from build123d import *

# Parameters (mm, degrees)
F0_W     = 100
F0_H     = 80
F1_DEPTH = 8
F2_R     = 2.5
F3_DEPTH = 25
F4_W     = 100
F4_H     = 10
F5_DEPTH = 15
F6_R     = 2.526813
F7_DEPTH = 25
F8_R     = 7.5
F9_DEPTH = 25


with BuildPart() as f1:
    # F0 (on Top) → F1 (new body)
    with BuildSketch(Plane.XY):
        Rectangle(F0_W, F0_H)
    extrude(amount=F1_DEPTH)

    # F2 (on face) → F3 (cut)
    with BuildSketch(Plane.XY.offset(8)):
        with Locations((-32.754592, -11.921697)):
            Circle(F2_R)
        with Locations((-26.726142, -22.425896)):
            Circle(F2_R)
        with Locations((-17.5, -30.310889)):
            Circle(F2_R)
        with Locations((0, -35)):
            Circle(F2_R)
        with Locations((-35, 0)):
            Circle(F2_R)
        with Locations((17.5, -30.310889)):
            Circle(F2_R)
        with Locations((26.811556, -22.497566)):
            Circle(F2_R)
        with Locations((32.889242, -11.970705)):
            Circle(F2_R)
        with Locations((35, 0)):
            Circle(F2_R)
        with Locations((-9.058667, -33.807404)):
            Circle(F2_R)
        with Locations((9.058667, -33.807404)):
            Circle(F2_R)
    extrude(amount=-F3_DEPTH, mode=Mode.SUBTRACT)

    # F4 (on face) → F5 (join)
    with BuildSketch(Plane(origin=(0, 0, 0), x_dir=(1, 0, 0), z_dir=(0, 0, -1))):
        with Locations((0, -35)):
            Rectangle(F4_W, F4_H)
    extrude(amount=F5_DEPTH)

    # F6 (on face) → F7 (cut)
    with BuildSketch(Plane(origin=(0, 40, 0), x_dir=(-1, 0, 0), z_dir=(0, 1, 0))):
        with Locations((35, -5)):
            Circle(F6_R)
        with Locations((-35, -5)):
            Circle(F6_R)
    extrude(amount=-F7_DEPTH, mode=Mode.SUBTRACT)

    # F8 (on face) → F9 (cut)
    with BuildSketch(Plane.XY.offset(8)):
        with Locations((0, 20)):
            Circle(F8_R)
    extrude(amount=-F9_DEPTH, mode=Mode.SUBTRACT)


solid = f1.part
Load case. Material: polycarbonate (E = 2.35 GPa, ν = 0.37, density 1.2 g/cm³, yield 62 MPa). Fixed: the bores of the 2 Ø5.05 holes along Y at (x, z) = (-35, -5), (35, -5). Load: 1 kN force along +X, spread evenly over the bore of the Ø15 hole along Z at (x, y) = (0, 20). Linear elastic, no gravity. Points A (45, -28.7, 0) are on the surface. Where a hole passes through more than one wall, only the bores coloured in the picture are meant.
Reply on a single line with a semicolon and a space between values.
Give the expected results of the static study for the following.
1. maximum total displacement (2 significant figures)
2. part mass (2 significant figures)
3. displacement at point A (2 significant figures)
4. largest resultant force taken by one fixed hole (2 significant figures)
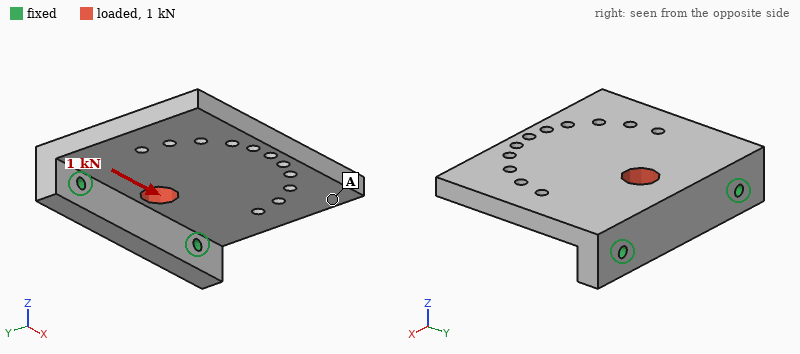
0.11 mm; 91 g; 0.099 mm; 550 N
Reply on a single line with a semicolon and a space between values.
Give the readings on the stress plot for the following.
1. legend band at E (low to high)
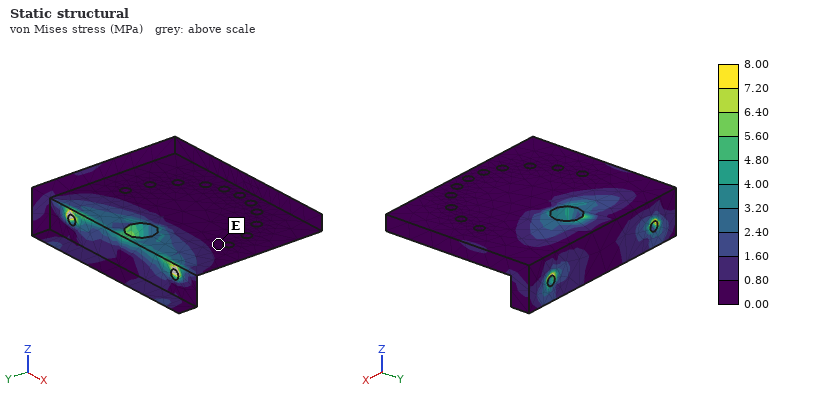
0.00 to 0.80 MPa
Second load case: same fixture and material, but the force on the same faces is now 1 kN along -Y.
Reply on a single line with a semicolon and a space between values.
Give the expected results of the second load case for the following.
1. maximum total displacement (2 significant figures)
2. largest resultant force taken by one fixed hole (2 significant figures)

0.49 mm; 510 N
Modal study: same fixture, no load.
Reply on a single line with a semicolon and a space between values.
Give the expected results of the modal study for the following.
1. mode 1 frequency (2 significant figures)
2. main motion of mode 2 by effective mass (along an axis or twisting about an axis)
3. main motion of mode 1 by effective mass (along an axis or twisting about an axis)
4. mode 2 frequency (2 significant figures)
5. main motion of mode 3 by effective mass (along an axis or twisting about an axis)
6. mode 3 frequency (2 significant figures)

280 Hz; twisting about Y; along Z; 580 Hz; along X; 1400 Hz
